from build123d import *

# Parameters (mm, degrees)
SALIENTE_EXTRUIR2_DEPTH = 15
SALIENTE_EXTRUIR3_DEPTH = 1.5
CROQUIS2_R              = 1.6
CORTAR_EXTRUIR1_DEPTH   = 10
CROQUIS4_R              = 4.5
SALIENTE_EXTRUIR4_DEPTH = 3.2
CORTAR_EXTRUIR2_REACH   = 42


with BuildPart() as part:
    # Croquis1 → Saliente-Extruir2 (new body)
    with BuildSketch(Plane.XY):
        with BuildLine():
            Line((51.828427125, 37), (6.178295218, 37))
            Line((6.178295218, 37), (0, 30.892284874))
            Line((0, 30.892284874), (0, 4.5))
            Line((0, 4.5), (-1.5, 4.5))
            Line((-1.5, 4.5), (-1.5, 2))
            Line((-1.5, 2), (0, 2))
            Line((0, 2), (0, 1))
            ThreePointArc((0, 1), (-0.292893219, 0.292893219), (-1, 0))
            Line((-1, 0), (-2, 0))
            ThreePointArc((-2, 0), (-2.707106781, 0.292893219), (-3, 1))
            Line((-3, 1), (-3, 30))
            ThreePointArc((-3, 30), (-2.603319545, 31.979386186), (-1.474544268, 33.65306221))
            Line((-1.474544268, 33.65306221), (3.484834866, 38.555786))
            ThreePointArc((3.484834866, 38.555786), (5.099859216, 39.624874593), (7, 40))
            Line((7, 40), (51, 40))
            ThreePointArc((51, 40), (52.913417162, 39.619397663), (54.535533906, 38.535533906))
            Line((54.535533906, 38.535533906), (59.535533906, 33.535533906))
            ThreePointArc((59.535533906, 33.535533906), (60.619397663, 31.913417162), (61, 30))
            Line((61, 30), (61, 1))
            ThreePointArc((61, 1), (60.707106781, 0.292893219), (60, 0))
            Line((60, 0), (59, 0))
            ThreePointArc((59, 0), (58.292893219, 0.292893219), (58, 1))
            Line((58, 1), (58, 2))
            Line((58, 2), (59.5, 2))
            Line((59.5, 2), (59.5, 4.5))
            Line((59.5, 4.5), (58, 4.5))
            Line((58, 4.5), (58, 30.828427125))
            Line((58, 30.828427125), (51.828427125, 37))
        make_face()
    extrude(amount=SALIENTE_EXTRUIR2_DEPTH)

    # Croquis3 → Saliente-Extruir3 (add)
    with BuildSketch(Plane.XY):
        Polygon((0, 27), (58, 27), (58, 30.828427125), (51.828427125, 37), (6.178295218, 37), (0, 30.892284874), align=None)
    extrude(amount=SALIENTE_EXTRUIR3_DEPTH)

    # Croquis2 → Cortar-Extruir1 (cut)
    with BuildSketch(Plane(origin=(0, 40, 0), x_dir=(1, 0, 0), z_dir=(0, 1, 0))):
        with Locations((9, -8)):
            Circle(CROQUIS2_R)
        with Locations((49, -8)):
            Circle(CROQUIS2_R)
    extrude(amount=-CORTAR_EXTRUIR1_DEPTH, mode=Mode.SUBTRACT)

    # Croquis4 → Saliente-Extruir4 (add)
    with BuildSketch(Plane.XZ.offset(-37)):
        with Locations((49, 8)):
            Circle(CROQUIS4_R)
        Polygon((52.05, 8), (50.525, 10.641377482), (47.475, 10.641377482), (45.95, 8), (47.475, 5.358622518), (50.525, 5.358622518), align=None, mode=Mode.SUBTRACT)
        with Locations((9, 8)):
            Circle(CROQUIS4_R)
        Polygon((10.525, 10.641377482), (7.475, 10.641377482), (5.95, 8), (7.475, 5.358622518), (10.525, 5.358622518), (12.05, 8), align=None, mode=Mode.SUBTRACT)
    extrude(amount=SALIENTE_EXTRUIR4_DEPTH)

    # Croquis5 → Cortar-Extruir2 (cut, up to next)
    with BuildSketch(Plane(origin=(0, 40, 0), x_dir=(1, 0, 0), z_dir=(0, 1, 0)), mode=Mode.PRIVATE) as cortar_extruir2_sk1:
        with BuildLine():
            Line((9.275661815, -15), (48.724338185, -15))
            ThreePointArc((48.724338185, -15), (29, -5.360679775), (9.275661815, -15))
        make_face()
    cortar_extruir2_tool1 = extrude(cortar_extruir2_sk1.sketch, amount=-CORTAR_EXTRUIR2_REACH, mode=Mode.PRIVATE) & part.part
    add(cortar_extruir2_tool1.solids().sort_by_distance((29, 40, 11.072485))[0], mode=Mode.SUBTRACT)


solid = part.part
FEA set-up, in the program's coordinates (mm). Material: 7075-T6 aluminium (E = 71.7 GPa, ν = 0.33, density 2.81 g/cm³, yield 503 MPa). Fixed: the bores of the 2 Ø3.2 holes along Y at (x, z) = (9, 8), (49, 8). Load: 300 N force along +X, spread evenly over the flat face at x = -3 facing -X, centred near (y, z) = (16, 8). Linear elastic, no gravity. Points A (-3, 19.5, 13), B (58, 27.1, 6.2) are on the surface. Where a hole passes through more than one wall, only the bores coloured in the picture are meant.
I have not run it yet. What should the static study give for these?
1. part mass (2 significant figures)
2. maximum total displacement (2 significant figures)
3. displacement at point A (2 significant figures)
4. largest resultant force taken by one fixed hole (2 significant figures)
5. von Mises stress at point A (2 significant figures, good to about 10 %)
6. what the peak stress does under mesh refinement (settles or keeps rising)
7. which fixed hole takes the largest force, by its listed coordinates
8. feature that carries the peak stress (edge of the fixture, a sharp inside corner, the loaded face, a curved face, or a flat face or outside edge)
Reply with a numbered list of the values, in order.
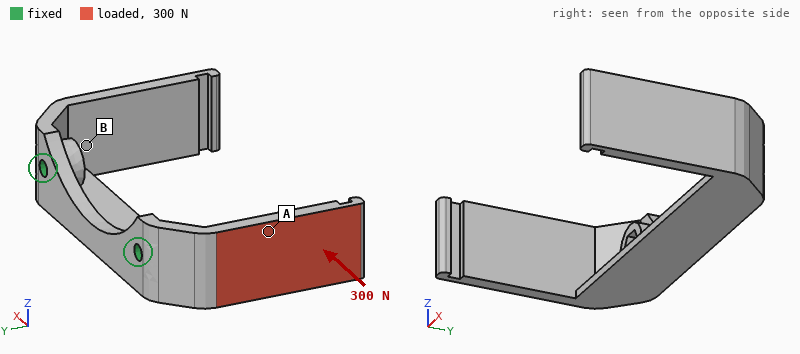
1. 17 g
2. 0.82 mm
3. 0.29 mm
4. 210 N
5. 76 MPa
6. keeps rising
7. (9, 8)
8. a sharp inside corner
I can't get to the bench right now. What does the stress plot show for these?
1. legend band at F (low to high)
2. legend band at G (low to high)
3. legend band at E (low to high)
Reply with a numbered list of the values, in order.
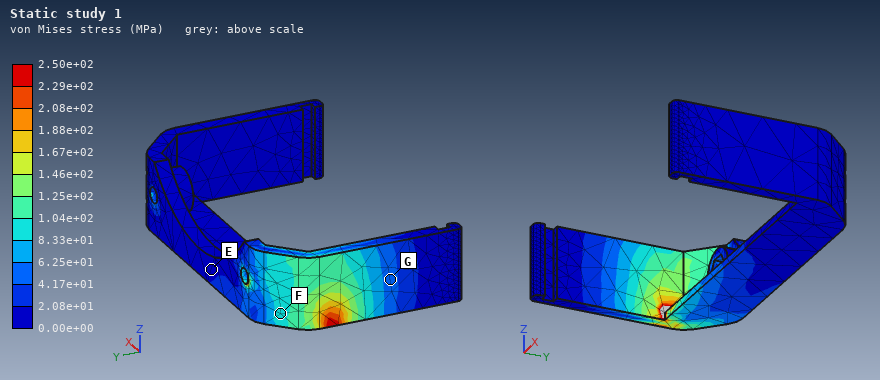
1. 8.33e+01 to 1.04e+02 MPa
2. 4.17e+01 to 6.25e+01 MPa
3. 0.00e+00 to 2.08e+01 MPa
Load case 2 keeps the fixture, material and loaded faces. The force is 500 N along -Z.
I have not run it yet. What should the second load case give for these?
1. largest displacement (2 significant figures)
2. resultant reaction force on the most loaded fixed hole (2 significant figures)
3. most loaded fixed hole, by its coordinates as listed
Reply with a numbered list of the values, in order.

1. 0.62 mm
2. 570 N
3. (9, 8)
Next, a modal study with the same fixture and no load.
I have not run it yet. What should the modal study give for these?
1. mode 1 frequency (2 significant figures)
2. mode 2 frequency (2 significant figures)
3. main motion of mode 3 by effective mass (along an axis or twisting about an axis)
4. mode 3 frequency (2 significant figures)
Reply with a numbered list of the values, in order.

1. 2100 Hz
2. 2100 Hz
3. twisting about Y
4. 2800 Hz
